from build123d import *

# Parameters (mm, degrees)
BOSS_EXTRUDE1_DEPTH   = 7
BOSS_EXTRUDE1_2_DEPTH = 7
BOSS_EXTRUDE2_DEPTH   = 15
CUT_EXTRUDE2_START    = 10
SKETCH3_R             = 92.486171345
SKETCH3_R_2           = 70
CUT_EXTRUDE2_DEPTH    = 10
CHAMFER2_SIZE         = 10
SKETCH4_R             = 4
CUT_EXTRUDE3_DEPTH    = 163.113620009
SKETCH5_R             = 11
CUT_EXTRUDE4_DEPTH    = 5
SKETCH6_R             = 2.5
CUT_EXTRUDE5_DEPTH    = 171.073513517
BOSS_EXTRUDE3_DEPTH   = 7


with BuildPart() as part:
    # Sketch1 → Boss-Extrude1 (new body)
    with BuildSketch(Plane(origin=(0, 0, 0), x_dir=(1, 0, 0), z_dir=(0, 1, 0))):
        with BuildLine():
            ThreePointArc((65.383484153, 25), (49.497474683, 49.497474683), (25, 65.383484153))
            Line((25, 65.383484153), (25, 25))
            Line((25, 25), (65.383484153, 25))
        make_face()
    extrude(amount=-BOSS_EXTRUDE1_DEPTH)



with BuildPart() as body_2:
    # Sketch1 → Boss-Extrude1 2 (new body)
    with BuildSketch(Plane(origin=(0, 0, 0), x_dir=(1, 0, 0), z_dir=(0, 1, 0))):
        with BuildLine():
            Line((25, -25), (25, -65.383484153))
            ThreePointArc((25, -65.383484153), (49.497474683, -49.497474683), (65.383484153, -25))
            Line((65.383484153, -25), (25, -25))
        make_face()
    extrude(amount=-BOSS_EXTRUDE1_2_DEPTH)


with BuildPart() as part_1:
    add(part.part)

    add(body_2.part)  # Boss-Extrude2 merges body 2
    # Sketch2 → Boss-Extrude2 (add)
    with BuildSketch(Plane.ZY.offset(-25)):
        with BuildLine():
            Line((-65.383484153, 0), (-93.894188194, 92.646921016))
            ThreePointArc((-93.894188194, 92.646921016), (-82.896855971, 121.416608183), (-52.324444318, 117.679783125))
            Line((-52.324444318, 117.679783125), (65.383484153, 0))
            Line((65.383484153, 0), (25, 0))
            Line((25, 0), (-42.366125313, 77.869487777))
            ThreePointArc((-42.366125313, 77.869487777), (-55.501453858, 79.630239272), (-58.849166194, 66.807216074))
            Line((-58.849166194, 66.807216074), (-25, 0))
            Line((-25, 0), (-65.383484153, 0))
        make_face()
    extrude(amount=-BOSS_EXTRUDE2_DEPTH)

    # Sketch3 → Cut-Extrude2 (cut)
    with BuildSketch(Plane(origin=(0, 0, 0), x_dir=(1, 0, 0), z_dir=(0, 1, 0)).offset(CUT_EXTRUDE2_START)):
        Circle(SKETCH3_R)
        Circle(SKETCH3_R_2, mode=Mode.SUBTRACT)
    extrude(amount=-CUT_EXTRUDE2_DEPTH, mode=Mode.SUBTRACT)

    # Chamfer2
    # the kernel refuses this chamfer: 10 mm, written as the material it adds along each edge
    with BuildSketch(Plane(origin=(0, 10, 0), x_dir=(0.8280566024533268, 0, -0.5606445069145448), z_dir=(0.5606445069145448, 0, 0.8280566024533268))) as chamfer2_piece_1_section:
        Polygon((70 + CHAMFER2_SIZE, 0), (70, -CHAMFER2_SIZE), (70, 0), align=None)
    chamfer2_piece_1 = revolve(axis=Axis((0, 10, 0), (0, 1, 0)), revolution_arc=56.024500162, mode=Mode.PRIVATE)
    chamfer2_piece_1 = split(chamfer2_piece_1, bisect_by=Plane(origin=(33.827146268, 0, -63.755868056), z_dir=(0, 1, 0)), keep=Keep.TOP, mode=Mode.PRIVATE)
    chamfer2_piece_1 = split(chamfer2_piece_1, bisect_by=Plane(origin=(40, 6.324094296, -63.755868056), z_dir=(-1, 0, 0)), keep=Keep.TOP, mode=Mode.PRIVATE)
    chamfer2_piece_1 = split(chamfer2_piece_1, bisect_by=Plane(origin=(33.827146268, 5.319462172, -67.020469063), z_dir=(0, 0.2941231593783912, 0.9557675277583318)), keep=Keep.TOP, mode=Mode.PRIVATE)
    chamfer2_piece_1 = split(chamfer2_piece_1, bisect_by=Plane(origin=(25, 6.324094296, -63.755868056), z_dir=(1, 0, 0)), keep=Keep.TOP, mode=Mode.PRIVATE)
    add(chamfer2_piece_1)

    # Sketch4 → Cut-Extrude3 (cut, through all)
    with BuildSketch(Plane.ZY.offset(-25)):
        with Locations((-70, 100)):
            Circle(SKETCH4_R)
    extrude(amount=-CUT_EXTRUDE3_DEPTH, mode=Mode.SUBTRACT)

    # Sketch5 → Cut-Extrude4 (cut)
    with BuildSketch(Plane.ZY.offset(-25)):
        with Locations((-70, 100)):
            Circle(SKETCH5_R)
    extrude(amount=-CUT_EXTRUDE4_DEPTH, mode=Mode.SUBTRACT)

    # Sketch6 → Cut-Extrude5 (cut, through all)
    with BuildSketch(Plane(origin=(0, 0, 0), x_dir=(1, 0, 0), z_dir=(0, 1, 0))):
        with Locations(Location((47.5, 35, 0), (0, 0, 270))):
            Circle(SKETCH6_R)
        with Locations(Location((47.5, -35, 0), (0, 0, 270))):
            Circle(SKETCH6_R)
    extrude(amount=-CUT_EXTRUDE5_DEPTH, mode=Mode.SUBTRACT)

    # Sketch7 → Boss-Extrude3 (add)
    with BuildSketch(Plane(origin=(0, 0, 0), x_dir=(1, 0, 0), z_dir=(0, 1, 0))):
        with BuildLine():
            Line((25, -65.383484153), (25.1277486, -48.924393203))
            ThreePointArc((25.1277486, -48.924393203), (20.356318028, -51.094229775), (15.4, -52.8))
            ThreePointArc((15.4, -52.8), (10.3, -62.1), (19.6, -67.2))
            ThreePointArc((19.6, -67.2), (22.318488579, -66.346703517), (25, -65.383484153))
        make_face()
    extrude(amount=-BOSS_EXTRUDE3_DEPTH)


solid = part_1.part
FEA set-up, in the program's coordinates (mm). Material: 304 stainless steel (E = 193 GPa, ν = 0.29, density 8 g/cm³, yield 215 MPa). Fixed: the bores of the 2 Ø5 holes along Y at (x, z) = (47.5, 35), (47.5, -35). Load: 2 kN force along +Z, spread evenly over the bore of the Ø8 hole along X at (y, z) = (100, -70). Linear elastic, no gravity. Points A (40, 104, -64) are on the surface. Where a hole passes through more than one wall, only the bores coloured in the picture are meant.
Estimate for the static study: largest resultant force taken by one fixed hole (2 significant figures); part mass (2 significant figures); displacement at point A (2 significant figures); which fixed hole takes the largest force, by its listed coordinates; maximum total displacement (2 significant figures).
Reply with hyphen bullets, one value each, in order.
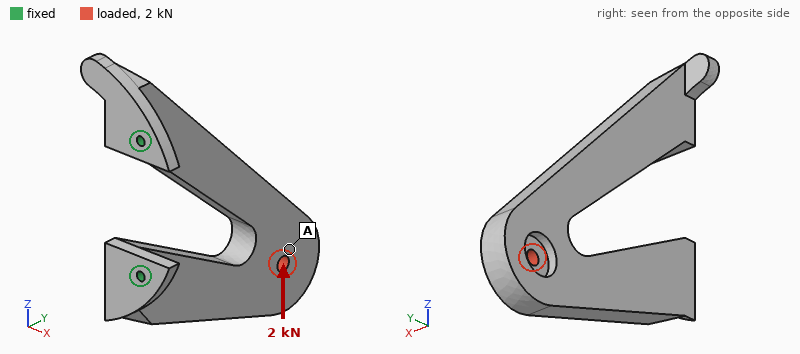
- 3.3 kN
- 1.0 kg
- 0.099 mm
- (47.5, 35)
- 0.11 mm
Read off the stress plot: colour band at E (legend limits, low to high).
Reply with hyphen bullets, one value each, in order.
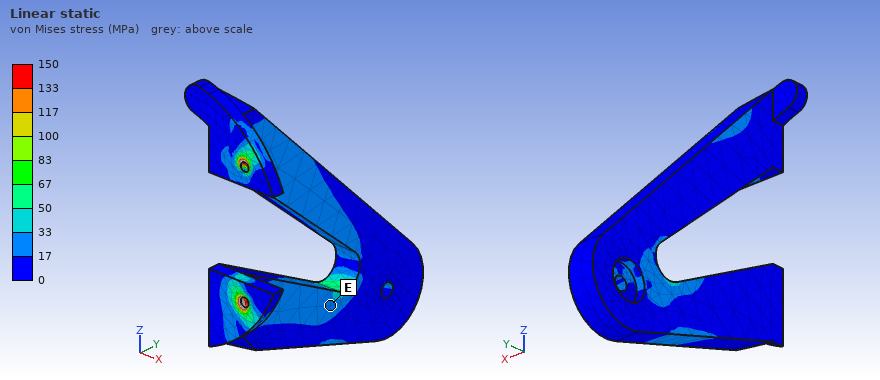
- 17 to 33 MPa
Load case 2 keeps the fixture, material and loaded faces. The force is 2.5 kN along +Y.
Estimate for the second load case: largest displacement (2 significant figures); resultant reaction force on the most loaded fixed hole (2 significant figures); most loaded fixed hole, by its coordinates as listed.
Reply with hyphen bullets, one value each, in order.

- 0.15 mm
- 3.5 kN
- (47.5, -35)
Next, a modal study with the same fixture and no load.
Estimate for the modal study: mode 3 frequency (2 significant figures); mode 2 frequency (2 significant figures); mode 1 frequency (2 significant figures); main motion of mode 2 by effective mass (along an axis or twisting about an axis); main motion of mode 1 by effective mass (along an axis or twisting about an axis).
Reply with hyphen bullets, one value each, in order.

- 1500 Hz
- 1000 Hz
- 320 Hz
- along Z
- along X
